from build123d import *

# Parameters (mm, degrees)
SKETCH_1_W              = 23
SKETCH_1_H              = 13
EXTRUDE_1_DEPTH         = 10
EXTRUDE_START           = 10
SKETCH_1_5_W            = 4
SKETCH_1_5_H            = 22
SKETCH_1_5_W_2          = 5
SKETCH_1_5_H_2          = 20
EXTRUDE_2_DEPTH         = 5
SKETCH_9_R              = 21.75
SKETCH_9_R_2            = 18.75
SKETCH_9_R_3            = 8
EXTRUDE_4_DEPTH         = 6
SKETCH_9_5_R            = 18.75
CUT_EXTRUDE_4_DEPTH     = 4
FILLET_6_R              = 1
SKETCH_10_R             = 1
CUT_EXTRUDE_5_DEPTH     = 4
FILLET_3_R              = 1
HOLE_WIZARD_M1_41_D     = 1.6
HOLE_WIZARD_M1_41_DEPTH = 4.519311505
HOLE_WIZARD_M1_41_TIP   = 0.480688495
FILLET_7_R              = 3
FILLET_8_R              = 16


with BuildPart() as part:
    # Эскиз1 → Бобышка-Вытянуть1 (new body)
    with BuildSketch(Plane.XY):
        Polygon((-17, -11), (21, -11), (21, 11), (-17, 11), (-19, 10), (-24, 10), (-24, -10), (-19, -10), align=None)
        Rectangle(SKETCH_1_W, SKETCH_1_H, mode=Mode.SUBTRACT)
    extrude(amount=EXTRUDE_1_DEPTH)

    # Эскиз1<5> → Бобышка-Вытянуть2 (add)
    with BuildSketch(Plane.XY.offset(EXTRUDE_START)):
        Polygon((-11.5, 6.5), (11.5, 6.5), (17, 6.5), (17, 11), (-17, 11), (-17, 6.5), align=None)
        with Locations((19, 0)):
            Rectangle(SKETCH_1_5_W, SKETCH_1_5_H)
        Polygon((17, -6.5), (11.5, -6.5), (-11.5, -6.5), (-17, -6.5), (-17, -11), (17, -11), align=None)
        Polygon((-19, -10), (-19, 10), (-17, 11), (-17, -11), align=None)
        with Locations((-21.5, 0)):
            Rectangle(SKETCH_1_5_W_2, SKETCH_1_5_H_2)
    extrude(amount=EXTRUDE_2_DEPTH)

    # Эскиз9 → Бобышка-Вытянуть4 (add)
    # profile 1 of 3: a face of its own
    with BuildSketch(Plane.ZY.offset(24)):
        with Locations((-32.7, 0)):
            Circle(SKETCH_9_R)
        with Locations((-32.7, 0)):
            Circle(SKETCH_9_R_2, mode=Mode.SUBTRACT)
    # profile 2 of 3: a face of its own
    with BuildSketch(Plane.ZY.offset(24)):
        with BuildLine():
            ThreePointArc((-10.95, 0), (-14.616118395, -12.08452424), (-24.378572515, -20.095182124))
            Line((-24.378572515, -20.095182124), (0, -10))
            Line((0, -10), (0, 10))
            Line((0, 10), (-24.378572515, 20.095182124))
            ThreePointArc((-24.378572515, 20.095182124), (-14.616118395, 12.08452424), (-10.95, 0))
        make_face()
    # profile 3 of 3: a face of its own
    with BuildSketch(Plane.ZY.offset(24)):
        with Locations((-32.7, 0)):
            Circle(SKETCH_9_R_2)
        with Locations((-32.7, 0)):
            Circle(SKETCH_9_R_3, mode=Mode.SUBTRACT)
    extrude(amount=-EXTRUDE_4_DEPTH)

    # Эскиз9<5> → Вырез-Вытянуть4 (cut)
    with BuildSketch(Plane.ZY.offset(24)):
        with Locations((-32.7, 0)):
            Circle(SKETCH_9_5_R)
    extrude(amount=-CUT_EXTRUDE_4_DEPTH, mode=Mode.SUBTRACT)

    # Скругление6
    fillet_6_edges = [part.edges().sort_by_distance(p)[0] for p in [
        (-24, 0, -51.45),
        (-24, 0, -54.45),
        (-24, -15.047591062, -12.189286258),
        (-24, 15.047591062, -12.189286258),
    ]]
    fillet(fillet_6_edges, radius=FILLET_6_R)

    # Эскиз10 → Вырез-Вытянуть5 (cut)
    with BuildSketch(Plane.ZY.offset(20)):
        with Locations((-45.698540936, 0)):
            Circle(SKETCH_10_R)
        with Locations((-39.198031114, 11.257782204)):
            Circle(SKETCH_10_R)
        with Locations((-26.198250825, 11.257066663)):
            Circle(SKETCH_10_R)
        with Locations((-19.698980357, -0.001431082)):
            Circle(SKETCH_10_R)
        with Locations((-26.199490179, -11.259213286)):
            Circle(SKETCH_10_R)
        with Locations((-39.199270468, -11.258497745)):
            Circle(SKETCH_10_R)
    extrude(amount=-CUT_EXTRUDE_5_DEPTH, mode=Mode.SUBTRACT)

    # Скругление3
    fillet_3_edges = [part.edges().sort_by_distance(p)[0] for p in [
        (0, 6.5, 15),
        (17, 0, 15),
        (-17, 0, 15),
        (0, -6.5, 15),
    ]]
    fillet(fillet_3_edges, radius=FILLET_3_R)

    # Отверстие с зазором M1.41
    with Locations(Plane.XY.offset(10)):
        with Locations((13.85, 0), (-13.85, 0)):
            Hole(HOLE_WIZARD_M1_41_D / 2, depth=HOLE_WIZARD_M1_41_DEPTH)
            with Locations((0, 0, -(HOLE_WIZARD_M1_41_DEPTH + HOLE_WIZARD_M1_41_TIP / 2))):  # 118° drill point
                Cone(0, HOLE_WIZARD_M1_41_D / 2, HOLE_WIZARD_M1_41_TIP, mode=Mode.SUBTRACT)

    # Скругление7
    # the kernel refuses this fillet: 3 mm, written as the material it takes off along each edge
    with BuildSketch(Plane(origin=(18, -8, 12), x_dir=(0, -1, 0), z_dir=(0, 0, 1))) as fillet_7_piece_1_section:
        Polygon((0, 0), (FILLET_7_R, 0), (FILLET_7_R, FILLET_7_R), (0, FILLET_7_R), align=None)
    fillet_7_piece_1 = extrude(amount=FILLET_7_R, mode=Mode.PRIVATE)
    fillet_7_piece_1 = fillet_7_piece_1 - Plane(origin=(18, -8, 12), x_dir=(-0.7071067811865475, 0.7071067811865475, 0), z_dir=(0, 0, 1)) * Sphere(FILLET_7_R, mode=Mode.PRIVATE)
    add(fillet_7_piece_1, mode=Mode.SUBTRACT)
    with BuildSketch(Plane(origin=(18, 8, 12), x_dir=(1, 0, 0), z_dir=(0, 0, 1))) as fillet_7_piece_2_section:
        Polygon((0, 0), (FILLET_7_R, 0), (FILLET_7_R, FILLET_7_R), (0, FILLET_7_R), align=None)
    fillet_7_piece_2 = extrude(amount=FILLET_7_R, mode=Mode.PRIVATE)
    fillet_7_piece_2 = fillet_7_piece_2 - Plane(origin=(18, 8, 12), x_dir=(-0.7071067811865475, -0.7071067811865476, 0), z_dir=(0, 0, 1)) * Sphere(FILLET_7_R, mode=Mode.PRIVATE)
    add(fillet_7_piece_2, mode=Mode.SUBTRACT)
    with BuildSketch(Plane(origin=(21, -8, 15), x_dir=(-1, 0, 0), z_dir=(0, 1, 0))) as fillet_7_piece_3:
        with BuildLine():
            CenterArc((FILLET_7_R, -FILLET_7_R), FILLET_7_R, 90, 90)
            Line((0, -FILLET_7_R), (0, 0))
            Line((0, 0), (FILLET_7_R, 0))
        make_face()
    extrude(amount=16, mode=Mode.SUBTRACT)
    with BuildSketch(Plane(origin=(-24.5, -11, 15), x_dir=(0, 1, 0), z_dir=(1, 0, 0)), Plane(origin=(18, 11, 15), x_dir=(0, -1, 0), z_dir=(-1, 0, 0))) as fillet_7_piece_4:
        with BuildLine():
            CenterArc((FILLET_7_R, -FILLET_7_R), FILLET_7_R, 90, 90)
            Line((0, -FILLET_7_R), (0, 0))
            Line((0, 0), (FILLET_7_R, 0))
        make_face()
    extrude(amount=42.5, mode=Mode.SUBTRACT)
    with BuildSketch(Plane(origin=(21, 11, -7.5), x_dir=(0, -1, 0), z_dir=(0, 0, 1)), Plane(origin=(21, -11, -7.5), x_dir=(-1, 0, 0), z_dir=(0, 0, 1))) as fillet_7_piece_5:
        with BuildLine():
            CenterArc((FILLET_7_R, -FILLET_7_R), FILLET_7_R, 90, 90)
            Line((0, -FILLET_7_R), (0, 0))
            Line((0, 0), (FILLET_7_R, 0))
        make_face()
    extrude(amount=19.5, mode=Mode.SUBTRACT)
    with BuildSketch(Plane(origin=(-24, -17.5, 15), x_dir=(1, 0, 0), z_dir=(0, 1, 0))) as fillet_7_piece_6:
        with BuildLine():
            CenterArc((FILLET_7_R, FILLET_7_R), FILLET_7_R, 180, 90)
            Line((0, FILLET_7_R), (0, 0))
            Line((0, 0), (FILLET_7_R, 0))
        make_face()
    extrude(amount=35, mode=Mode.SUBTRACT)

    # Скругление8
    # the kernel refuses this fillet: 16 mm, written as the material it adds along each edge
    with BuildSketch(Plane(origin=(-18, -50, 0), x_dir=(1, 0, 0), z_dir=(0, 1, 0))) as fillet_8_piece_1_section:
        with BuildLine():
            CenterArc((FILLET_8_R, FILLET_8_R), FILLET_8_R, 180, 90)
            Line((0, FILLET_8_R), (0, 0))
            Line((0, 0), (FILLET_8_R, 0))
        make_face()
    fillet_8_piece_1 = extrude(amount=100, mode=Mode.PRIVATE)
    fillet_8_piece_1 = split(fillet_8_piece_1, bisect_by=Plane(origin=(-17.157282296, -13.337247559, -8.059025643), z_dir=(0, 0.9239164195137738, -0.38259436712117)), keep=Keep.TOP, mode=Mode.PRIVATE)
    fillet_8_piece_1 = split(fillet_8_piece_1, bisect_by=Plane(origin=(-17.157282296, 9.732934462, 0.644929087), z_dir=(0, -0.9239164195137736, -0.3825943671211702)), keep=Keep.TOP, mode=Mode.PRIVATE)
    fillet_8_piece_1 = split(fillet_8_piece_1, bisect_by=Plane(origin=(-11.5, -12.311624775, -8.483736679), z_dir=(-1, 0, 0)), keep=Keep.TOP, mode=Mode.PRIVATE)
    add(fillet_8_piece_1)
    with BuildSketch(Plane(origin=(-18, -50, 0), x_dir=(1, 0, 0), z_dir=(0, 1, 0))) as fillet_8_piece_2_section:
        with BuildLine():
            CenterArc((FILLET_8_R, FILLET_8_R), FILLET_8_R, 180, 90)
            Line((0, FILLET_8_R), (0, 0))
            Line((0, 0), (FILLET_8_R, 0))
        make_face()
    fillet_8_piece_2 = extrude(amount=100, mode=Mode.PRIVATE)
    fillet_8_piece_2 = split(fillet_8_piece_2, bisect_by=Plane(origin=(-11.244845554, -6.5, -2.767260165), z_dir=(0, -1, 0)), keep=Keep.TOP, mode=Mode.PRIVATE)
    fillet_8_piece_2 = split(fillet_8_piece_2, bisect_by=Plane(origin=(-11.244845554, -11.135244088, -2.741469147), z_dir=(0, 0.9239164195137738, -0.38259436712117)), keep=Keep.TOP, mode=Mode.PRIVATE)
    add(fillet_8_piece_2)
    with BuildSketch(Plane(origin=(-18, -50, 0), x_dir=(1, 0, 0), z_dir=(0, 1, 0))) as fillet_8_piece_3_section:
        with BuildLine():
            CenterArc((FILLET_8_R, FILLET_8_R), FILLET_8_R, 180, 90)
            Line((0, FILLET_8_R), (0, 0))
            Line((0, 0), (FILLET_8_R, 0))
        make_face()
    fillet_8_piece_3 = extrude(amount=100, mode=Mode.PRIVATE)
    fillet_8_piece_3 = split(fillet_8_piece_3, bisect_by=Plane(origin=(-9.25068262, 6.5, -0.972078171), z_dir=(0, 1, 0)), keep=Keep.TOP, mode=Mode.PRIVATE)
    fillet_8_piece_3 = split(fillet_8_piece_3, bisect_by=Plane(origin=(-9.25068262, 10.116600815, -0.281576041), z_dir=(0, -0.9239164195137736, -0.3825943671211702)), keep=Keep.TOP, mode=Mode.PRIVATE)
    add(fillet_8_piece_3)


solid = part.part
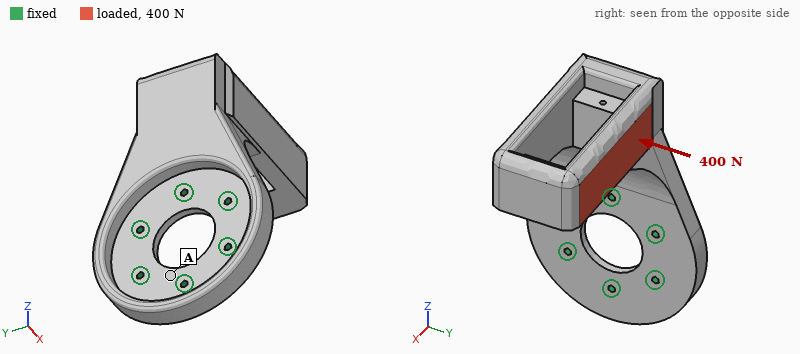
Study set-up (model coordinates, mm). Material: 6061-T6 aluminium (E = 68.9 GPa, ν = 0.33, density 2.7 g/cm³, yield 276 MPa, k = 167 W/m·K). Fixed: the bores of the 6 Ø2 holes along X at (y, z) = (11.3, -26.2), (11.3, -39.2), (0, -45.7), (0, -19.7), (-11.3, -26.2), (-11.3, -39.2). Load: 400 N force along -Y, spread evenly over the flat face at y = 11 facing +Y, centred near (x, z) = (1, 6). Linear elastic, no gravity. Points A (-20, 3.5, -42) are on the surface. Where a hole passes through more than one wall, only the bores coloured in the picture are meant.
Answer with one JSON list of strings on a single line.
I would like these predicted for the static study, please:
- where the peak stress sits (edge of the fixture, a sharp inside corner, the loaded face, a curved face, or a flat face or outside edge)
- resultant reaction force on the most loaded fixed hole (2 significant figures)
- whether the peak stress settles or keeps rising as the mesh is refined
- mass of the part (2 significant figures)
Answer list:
["edge of the fixture", "410 N", "keeps rising", "44 g"]
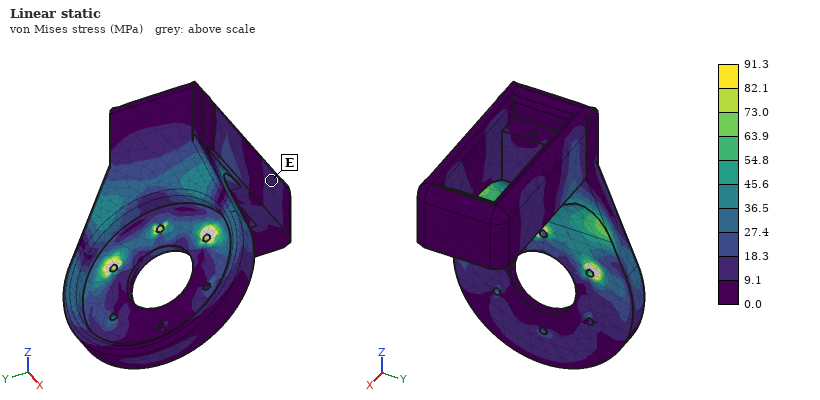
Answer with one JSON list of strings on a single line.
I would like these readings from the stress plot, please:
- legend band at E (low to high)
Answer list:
["9.1 to 18.3 MPa"]
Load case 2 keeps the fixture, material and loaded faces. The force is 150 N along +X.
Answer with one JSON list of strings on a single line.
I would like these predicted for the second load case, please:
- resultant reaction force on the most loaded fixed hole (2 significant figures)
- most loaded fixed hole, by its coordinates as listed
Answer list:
["360 N", "(0, -19.7)"]
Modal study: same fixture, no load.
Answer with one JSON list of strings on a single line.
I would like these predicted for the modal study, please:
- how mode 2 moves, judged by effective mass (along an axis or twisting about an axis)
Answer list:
["along Y"]
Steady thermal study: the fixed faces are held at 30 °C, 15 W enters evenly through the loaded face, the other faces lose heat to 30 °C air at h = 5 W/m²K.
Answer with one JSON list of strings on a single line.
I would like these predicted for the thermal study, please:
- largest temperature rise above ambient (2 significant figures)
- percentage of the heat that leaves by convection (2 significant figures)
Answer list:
["30 K", "3.5 %"]
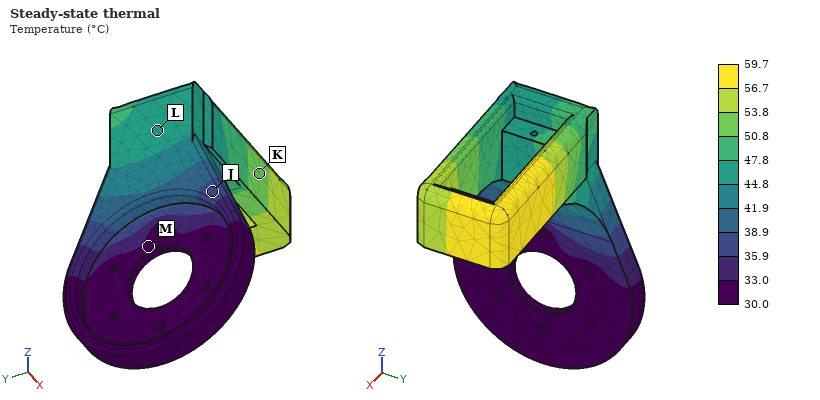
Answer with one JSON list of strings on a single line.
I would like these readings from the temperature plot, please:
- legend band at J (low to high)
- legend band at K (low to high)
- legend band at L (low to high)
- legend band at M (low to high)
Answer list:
["35.9 to 38.9 °C", "50.8 to 53.8 °C", "44.8 to 47.8 °C", "30.0 to 33.0 °C"]
